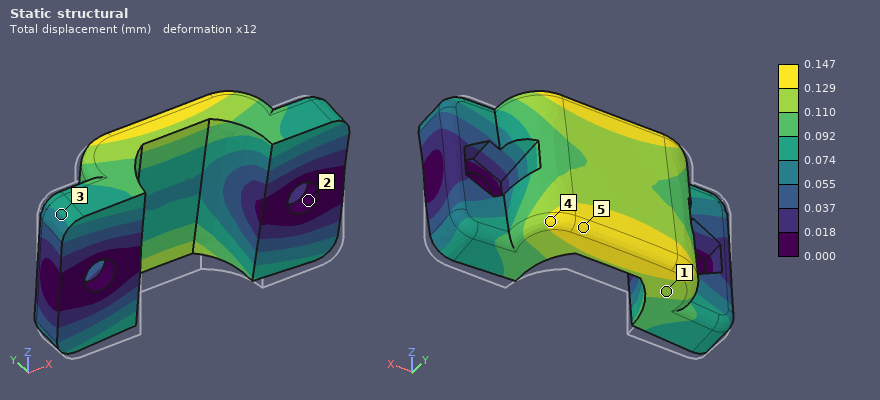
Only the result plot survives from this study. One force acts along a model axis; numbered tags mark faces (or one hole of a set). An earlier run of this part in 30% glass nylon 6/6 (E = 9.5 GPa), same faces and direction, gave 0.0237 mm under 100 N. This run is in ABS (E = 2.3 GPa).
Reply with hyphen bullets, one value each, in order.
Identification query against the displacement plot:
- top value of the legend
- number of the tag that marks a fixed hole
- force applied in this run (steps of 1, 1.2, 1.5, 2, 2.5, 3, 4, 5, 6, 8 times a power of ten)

- 0.147 mm
- 2
- 150 N
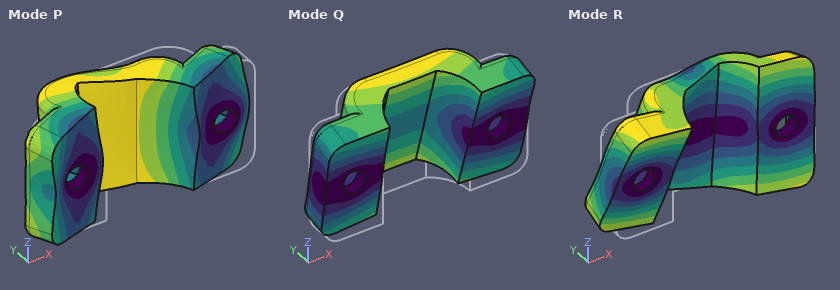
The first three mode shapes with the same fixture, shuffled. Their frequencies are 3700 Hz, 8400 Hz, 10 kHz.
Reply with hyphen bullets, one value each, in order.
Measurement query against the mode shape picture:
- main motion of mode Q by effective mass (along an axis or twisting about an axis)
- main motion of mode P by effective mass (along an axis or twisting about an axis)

- along Z
- along X
